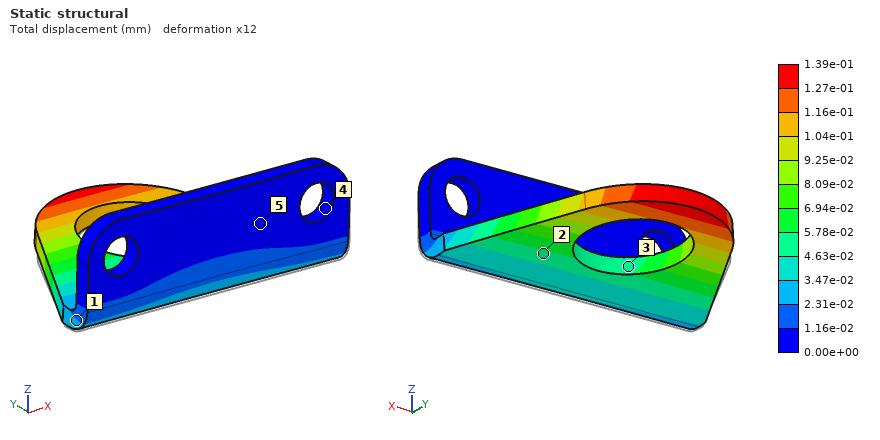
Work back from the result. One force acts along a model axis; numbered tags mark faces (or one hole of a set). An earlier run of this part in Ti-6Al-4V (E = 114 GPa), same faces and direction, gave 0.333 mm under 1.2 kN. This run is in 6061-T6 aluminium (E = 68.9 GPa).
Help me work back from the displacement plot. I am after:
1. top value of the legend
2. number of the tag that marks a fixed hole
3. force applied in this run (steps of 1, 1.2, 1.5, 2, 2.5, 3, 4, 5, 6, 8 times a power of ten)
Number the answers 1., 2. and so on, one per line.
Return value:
1. 1.39e-01 mm
2. 4
3. 300 N
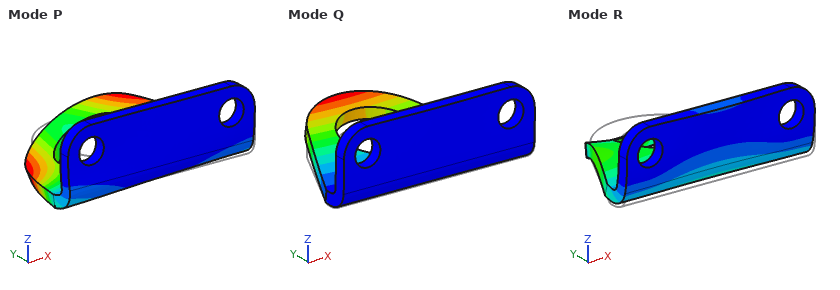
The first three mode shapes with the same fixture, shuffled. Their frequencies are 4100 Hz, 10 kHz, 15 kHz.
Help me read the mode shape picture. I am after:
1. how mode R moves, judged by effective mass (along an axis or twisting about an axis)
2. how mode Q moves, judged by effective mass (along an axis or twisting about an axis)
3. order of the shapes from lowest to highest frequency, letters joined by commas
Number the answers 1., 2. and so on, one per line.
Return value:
1. along Y
2. along Z
3. Q, P, R
